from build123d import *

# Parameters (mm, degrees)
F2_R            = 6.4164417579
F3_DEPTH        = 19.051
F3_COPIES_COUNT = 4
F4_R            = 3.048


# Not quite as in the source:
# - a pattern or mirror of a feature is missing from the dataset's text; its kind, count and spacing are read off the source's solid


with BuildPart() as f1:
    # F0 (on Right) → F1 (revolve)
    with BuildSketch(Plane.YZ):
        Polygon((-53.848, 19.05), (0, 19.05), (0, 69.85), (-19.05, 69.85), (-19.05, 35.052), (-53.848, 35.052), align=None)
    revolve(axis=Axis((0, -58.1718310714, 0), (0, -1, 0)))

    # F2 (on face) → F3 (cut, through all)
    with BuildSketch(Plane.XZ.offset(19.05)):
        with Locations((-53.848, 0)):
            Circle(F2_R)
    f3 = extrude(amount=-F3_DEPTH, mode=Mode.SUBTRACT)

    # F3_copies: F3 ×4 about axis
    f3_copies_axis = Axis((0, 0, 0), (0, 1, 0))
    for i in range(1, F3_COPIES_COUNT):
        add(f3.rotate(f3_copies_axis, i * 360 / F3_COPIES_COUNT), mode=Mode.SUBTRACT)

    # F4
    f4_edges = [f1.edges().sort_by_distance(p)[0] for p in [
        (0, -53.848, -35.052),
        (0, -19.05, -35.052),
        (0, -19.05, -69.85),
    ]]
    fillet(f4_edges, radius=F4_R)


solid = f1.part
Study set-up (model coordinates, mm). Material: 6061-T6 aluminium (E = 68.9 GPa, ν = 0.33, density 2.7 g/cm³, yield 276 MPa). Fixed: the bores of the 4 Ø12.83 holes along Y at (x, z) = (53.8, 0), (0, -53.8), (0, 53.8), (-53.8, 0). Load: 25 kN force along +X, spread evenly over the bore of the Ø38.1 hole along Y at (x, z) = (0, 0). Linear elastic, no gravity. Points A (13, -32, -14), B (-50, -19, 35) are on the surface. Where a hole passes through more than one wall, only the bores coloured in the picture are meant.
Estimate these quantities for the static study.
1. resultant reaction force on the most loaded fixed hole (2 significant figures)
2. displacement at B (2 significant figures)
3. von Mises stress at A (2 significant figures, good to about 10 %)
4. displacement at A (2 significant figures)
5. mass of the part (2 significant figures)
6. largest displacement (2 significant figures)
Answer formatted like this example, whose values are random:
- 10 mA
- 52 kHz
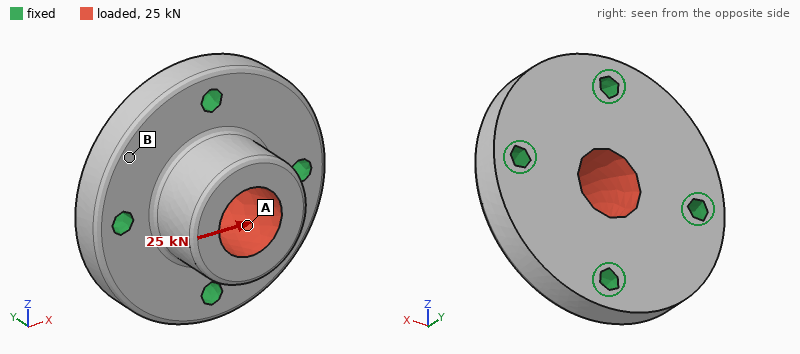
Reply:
- 9.0 kN
- 4.4 µm
- 11 MPa
- 12 µm
- 960 g
- 21 µm
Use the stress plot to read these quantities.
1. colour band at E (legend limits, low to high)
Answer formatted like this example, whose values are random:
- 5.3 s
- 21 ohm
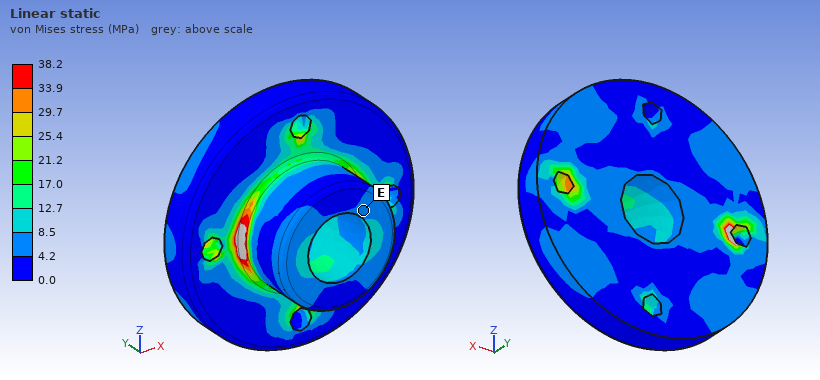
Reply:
- 4.2 to 8.5 MPa
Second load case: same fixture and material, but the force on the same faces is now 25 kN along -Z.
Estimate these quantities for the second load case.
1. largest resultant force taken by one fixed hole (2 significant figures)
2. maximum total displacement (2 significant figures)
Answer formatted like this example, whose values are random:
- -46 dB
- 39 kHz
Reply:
- 9.0 kN
- 21 µm
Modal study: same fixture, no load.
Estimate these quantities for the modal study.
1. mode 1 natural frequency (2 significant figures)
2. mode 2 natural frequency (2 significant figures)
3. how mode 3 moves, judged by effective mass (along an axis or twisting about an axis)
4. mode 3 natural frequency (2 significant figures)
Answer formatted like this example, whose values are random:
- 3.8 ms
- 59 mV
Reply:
- 9300 Hz
- 9300 Hz
- along Y
- 9700 Hz
